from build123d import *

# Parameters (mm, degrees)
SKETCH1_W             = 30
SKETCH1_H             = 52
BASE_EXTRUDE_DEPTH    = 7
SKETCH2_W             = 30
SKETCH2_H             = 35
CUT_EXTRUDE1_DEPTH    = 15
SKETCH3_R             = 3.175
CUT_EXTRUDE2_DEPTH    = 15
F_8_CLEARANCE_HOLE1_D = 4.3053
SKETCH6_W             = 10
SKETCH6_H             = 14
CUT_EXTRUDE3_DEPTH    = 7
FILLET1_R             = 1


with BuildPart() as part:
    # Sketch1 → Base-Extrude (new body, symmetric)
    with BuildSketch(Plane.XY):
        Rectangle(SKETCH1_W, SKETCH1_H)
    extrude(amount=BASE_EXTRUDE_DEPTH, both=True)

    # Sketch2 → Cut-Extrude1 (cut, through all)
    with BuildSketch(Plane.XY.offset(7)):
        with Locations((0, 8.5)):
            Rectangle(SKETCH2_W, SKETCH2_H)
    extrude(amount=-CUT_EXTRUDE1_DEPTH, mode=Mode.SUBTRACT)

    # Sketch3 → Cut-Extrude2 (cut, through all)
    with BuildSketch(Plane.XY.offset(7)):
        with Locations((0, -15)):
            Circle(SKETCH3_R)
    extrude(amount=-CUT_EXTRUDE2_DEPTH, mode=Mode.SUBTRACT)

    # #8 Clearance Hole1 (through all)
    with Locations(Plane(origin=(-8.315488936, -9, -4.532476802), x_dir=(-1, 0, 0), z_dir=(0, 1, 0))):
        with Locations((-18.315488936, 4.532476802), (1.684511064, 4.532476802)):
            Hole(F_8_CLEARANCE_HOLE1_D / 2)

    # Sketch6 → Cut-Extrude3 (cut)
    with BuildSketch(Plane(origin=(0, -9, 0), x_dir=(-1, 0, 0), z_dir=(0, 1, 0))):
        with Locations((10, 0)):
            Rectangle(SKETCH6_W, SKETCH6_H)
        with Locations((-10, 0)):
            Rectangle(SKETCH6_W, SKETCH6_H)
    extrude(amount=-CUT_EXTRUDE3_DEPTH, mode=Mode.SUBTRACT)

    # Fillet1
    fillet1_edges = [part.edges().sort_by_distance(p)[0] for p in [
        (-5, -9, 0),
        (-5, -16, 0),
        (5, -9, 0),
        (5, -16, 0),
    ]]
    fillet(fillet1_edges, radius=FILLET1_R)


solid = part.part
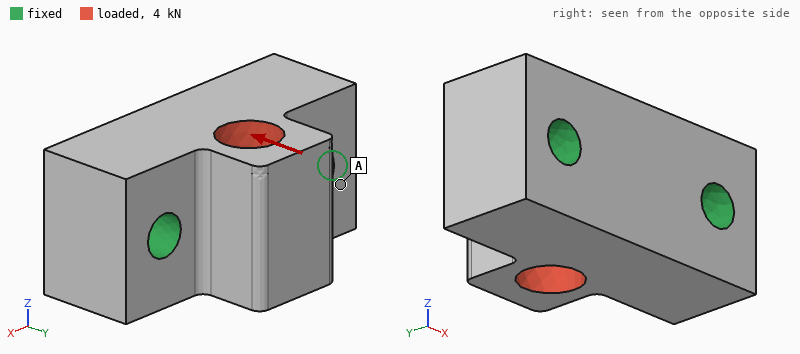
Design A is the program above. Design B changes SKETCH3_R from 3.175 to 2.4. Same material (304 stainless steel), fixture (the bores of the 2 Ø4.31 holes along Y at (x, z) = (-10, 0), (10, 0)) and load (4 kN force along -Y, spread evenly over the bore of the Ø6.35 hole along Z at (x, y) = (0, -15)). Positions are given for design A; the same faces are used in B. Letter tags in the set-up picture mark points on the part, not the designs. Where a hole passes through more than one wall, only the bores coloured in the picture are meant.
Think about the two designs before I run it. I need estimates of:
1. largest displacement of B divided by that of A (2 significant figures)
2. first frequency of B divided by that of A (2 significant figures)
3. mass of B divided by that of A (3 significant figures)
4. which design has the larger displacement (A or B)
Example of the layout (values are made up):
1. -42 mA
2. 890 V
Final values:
1. 0.89
2. 0.99
3. 1.04
4. A
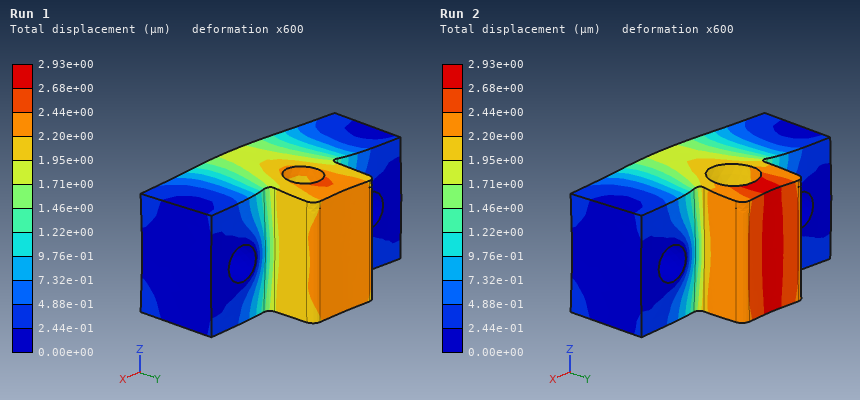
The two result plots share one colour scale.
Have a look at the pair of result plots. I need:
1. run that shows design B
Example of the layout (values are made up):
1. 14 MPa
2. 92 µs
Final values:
1. Run 1
